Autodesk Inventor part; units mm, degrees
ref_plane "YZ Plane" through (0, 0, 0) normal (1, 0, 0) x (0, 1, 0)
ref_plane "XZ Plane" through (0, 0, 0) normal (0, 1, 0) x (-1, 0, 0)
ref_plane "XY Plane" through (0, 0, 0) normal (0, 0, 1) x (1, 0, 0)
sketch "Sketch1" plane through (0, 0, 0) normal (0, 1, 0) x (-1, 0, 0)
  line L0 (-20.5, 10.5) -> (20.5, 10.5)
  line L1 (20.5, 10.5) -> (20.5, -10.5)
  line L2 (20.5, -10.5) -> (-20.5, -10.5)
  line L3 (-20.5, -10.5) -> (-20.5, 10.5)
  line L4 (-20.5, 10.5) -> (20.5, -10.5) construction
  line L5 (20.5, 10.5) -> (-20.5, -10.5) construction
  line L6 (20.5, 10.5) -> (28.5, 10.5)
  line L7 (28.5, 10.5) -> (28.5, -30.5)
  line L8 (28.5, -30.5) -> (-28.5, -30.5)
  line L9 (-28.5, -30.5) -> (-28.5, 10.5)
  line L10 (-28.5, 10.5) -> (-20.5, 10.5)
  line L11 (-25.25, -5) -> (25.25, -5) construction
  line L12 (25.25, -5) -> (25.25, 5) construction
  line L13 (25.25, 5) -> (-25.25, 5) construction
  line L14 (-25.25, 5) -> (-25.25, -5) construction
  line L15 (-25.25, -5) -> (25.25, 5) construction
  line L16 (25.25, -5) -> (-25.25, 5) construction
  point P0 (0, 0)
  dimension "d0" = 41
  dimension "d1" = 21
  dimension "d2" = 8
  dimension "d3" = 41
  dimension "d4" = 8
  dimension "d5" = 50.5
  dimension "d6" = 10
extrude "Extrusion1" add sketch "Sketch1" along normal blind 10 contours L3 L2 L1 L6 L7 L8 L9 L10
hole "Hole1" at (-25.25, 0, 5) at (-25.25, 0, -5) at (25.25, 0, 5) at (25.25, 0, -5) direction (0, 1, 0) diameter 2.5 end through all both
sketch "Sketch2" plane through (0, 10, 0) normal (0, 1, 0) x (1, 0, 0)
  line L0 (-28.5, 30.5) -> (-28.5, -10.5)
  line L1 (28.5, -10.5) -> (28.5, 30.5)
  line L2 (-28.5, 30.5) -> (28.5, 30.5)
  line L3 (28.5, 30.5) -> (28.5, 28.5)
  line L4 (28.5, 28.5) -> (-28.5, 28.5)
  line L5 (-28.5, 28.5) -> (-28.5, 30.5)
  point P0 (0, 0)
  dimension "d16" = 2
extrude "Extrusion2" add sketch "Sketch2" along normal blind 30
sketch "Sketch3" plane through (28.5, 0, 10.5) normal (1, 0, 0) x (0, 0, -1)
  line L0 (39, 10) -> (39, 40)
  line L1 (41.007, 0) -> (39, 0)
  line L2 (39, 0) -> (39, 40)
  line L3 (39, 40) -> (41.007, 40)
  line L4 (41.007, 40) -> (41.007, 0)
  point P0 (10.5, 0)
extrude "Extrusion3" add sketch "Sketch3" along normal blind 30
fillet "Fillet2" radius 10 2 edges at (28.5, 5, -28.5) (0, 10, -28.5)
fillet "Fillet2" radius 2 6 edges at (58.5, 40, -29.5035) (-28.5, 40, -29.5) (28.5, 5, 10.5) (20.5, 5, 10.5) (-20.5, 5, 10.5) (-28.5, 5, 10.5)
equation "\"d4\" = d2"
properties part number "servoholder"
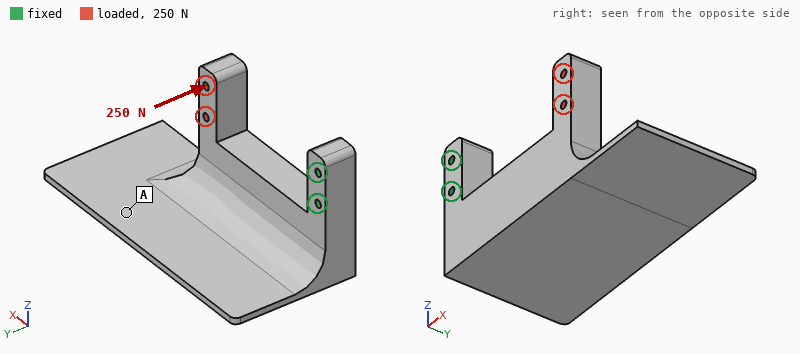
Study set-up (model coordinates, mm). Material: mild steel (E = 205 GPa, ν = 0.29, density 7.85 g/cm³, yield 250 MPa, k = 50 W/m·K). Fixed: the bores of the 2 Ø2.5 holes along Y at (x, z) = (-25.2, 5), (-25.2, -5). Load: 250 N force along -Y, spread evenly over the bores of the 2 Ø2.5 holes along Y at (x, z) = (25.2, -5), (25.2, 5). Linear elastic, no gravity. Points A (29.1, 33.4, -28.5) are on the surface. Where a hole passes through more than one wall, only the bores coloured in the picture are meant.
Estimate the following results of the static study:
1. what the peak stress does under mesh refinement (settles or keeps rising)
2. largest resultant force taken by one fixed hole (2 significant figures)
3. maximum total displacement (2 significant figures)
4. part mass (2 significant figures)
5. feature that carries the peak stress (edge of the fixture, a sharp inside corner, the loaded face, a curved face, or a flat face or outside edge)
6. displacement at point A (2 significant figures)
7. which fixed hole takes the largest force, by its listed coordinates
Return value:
keeps rising
170 N
0.15 mm
170 g
edge of the fixture
0.10 mm
(-25.2, -5)
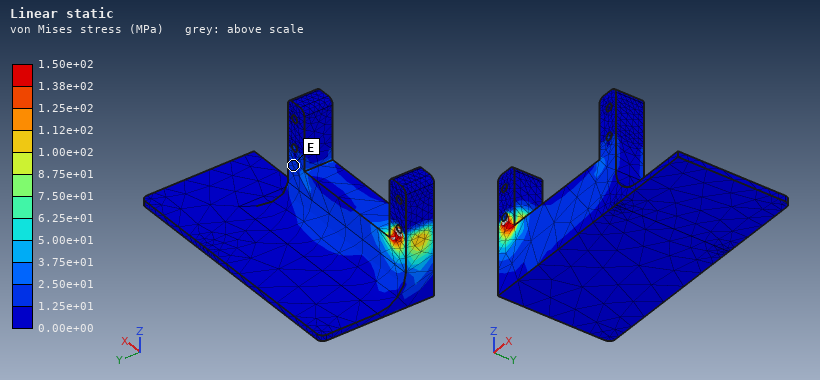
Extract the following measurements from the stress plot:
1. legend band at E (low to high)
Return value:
1.25e+01 to 2.50e+01 MPa
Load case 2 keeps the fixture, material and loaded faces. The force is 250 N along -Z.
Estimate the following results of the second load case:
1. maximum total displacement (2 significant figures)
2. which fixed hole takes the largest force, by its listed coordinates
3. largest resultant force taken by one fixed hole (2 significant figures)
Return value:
0.16 mm
(-25.2, 5)
790 N
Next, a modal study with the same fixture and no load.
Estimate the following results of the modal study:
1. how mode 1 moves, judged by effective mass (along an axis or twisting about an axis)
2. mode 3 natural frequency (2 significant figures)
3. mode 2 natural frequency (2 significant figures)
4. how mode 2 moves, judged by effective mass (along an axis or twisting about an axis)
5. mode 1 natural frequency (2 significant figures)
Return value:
along Z
2000 Hz
830 Hz
along Y
770 Hz
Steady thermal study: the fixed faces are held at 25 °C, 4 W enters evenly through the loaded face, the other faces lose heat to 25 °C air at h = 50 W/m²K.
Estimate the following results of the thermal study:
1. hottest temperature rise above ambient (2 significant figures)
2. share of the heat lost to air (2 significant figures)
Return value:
23 K
75 %
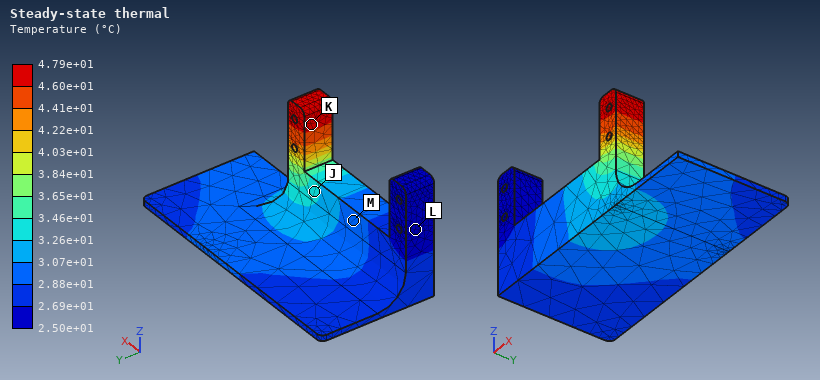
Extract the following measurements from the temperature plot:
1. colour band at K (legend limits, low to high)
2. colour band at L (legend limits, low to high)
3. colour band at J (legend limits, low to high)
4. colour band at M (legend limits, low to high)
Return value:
4.60e+01 to 4.79e+01 °C
2.50e+01 to 2.69e+01 °C
3.26e+01 to 3.46e+01 °C
2.88e+01 to 3.07e+01 °C
